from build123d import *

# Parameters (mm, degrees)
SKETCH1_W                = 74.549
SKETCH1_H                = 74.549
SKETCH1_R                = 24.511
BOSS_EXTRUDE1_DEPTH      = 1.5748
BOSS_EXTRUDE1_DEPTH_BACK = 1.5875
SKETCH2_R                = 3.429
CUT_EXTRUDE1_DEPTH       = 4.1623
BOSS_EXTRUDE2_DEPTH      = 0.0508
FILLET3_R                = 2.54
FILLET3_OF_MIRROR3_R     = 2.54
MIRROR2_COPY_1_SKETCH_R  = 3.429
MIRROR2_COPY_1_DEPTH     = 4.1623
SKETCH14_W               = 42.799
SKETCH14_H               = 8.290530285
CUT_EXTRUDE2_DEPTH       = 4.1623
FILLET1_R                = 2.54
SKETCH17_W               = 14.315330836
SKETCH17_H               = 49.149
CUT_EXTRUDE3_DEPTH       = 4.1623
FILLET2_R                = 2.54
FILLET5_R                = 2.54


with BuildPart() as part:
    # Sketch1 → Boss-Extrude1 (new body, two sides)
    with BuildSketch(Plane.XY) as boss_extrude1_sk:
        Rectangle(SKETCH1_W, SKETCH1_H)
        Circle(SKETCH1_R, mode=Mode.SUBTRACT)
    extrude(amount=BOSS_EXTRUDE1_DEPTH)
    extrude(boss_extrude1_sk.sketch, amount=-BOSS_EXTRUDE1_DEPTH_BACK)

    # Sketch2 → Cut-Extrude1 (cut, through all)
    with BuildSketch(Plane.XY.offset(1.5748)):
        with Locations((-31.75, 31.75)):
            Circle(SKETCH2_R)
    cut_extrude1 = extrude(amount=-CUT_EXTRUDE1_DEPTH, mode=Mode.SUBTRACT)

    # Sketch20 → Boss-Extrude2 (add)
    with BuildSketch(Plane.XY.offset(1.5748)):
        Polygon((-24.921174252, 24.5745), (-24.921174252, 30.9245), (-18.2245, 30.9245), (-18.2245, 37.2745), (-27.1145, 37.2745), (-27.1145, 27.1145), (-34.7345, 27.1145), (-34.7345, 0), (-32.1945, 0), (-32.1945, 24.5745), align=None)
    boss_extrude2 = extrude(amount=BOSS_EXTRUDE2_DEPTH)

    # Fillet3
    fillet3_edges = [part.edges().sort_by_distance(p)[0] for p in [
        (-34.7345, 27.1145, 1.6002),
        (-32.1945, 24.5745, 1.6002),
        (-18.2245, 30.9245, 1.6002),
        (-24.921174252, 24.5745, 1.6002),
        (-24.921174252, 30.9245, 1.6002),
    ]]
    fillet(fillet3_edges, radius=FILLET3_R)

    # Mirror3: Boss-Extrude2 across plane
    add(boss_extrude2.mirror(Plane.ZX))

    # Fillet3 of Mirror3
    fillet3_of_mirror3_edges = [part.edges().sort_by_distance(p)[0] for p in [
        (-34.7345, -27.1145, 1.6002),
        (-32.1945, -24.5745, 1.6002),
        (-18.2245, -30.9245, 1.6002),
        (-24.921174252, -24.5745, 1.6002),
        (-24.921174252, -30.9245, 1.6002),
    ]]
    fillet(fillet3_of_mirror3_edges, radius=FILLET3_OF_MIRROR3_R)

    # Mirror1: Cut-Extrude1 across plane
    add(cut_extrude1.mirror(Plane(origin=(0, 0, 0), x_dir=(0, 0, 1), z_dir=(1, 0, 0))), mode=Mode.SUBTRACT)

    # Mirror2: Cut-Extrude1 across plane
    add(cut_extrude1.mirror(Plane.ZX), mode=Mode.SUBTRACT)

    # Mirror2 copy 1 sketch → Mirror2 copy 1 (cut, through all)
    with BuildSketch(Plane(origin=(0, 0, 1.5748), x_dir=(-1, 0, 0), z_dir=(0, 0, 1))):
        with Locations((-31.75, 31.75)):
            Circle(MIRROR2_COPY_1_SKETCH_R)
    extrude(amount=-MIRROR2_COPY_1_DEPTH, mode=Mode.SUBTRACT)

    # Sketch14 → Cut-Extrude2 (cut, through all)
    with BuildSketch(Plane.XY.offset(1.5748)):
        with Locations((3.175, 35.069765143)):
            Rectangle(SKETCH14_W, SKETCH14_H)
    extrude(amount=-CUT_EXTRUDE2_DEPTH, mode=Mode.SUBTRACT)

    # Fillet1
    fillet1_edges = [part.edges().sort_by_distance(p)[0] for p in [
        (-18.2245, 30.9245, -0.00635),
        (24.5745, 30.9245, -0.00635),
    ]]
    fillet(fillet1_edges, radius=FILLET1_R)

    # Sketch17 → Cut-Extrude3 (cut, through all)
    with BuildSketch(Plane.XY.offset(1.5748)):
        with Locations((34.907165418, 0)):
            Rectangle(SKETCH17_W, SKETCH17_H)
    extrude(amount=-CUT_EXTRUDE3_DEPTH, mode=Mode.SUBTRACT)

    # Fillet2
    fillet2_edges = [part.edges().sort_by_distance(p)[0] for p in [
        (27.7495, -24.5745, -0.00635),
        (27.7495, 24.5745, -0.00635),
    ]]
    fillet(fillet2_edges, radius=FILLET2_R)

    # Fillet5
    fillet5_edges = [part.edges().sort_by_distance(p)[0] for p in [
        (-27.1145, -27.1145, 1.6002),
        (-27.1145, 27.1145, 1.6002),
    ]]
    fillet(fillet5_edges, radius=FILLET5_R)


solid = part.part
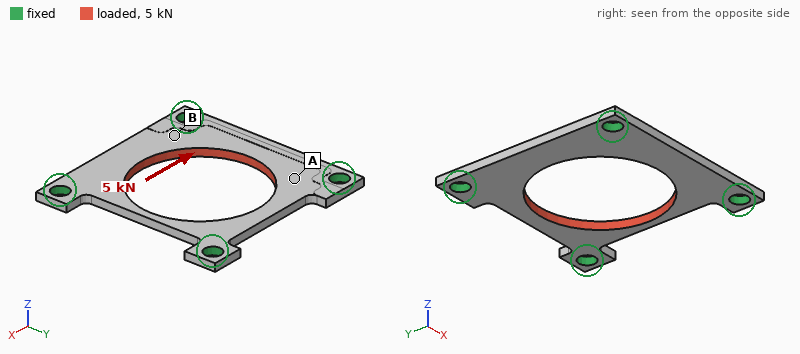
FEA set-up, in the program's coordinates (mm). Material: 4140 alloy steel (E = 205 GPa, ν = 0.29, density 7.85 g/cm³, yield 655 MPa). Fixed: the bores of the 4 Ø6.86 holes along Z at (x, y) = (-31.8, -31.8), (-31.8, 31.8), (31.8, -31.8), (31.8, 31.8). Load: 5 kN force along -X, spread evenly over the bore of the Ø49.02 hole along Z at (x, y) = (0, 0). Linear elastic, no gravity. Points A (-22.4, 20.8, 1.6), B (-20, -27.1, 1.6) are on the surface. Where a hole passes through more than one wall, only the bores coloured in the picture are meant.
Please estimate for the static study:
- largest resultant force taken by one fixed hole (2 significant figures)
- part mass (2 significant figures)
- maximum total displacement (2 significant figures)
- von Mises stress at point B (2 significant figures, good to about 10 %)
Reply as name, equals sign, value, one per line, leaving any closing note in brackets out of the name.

largest resultant force taken by one fixed hole = 1.4 kN
part mass = 69 g
maximum total displacement = 37 µm
von Mises stress at point B = 20 MPa
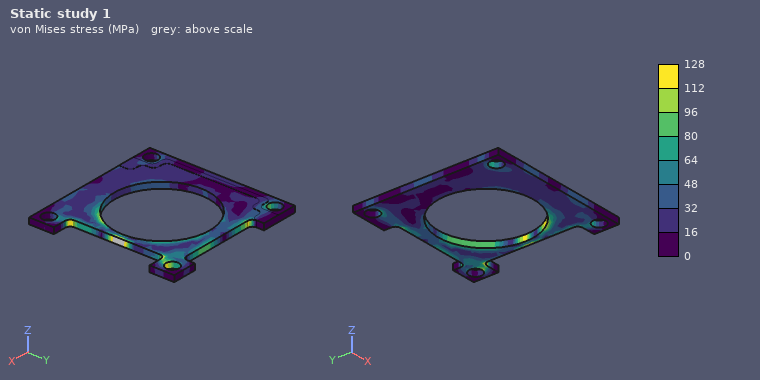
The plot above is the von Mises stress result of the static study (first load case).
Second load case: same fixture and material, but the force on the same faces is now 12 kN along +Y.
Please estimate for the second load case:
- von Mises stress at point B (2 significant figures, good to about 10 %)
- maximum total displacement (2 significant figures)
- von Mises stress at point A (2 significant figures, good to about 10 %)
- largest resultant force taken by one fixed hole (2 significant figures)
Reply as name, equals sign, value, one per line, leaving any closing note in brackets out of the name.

von Mises stress at point B = 50 MPa
maximum total displacement = 54 µm
von Mises stress at point A = 52 MPa
largest resultant force taken by one fixed hole = 3.6 kN
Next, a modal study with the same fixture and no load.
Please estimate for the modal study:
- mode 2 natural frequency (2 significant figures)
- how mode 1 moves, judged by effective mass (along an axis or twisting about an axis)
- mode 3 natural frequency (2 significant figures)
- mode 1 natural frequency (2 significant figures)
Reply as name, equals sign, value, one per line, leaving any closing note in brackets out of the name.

mode 2 natural frequency = 5000 Hz
how mode 1 moves, judged by effective mass = along Z
mode 3 natural frequency = 5300 Hz
mode 1 natural frequency = 4700 Hz
